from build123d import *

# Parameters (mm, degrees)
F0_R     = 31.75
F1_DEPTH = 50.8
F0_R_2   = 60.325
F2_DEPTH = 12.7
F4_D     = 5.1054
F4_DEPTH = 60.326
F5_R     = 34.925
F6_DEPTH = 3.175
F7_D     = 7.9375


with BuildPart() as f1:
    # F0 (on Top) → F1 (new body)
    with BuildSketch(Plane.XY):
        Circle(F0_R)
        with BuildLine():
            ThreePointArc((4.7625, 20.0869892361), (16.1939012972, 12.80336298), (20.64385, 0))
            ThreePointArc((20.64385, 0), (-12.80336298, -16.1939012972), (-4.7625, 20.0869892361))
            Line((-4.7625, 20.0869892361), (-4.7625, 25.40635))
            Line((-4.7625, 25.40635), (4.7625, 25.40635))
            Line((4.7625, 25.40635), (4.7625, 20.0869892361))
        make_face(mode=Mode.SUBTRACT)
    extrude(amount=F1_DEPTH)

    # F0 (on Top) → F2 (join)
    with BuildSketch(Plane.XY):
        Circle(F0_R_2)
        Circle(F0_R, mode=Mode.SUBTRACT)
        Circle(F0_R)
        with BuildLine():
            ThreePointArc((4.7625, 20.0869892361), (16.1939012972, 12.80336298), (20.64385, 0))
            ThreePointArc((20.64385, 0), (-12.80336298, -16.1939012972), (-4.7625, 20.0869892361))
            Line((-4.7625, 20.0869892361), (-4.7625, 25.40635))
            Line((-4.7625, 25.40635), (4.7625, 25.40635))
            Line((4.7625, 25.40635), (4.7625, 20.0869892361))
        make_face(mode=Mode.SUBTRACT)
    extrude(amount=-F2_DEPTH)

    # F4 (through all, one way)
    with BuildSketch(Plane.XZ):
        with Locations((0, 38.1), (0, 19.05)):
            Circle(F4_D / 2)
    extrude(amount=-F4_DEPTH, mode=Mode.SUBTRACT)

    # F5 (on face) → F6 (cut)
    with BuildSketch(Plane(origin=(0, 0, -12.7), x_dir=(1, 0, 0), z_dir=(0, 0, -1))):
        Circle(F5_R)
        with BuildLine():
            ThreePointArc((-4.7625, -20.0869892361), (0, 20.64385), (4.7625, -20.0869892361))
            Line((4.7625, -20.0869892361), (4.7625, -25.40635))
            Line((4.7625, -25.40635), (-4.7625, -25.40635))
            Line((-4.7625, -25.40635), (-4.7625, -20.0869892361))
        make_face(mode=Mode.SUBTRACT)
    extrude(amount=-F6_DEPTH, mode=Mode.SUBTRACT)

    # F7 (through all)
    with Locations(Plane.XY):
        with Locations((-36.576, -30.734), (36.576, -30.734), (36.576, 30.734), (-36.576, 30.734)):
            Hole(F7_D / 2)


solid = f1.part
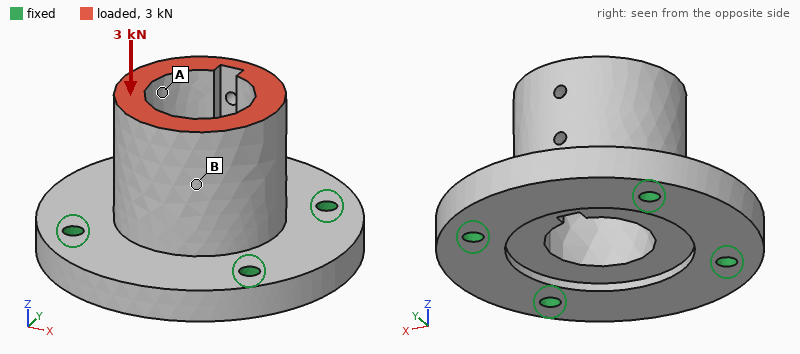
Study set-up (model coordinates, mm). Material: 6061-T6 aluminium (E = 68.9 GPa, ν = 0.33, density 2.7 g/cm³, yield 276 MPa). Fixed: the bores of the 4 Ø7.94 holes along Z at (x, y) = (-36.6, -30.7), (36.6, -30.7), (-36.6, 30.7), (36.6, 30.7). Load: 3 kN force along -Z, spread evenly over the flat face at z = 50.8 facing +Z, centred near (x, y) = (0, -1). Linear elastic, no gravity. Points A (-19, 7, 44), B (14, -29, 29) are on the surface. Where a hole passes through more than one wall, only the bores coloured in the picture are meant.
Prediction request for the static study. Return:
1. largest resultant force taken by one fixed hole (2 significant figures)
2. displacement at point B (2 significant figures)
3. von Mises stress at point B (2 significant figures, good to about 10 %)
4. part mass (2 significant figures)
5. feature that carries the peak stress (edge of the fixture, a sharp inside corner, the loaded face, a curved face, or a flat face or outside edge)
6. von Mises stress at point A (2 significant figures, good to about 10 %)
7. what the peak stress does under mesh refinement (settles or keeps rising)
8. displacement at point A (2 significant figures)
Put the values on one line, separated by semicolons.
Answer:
830 N; 4.5 µm; 1.4 MPa; 560 g; edge of the fixture; 2.1 MPa; keeps rising; 4.7 µm
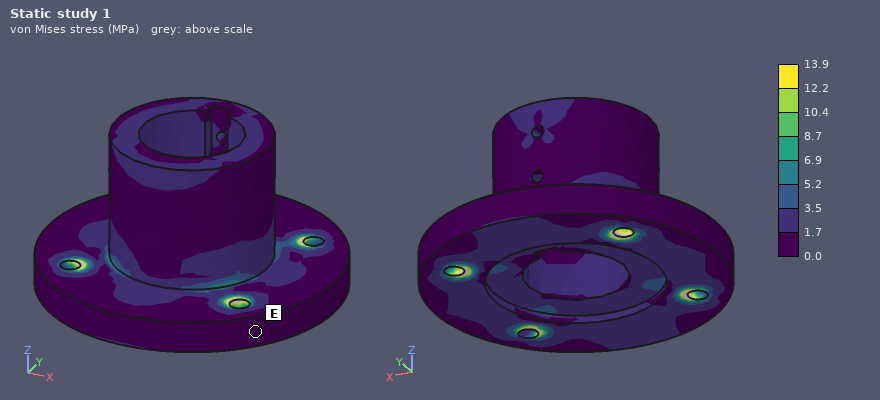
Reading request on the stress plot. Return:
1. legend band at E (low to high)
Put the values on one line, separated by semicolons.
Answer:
0.0 to 1.7 MPa
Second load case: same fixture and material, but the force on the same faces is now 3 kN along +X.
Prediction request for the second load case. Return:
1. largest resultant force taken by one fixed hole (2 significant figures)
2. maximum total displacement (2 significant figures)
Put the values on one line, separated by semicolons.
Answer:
1.6 kN; 27 µm
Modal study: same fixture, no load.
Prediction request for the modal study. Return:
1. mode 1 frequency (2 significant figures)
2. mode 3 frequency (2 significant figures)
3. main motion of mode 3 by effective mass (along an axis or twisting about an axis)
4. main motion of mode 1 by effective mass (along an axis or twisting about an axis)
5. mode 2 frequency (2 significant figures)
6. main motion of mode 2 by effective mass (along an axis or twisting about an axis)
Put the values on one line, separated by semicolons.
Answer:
5100 Hz; 7300 Hz; along Z; along Y; 5700 Hz; along X
